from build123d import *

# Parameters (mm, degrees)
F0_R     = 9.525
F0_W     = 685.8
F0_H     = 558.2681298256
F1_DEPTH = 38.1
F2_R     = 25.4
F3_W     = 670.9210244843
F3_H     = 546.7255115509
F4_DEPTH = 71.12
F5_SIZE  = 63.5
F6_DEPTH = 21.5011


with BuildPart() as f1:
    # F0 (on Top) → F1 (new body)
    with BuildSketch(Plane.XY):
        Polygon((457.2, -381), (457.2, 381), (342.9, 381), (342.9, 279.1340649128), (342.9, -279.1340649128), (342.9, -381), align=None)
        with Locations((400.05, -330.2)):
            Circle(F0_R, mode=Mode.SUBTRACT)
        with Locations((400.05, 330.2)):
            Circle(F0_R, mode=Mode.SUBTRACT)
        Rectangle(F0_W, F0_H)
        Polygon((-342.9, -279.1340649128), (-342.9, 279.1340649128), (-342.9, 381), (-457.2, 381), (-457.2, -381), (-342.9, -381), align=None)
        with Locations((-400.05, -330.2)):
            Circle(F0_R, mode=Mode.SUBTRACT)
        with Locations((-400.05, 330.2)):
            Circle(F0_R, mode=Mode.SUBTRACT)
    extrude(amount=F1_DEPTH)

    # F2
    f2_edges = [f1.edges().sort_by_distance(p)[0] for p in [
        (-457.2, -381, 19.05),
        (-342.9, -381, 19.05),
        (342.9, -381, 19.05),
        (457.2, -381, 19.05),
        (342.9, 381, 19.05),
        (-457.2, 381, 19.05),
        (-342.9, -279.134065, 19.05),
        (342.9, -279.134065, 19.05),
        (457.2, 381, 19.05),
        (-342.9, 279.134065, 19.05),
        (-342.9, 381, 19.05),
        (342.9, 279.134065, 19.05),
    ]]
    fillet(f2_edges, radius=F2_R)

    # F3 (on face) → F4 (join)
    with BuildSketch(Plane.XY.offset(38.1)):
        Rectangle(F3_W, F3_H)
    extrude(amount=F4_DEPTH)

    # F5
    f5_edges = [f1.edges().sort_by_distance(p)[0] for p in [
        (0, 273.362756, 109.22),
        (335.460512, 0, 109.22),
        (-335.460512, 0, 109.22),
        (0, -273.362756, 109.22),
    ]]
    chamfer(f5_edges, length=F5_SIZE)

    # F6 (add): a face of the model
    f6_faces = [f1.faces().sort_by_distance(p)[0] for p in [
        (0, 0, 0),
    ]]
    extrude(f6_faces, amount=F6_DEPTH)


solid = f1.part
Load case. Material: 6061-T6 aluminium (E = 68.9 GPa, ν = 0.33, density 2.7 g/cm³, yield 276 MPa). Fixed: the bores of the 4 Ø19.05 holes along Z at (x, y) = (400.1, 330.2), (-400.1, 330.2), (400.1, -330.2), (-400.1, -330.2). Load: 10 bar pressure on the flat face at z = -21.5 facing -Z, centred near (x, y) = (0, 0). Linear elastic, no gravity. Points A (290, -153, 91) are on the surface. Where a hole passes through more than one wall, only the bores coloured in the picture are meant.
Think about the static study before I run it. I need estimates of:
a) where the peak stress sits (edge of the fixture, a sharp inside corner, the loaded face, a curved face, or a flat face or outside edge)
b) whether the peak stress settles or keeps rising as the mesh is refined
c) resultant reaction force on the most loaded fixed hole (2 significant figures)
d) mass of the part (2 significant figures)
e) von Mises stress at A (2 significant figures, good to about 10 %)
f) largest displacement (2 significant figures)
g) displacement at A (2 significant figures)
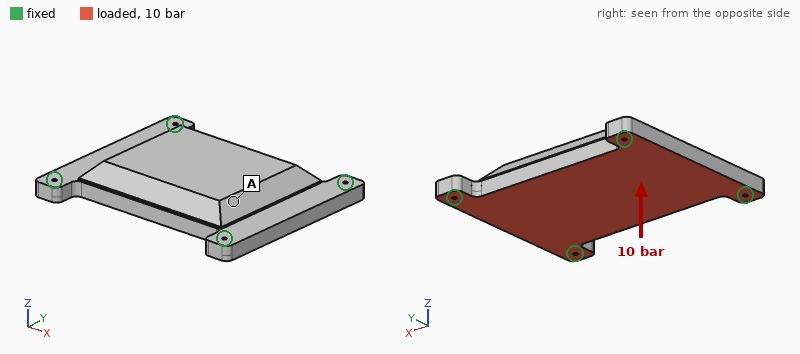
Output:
edge of the fixture
keeps rising
160 kN
150 kg
30 MPa
0.75 mm
0.57 mm
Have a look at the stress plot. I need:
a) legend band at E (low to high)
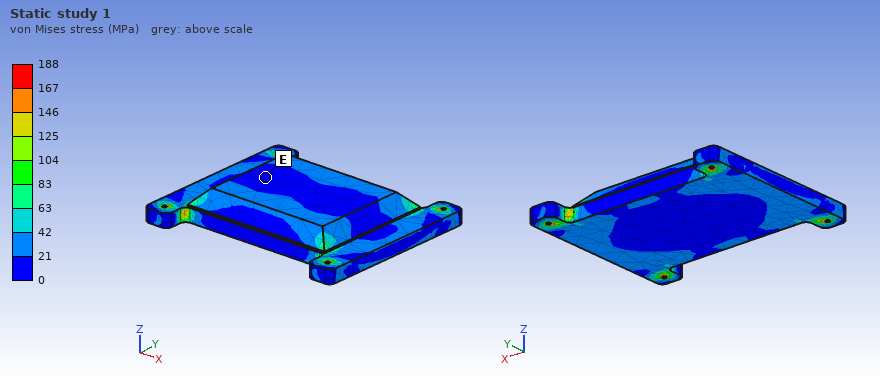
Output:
0 to 21 MPa
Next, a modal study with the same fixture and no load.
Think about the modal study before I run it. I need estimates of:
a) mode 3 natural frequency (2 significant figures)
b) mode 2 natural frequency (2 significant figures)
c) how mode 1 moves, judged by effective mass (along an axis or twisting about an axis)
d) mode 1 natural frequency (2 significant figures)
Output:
690 Hz
670 Hz
along Z
360 Hz
